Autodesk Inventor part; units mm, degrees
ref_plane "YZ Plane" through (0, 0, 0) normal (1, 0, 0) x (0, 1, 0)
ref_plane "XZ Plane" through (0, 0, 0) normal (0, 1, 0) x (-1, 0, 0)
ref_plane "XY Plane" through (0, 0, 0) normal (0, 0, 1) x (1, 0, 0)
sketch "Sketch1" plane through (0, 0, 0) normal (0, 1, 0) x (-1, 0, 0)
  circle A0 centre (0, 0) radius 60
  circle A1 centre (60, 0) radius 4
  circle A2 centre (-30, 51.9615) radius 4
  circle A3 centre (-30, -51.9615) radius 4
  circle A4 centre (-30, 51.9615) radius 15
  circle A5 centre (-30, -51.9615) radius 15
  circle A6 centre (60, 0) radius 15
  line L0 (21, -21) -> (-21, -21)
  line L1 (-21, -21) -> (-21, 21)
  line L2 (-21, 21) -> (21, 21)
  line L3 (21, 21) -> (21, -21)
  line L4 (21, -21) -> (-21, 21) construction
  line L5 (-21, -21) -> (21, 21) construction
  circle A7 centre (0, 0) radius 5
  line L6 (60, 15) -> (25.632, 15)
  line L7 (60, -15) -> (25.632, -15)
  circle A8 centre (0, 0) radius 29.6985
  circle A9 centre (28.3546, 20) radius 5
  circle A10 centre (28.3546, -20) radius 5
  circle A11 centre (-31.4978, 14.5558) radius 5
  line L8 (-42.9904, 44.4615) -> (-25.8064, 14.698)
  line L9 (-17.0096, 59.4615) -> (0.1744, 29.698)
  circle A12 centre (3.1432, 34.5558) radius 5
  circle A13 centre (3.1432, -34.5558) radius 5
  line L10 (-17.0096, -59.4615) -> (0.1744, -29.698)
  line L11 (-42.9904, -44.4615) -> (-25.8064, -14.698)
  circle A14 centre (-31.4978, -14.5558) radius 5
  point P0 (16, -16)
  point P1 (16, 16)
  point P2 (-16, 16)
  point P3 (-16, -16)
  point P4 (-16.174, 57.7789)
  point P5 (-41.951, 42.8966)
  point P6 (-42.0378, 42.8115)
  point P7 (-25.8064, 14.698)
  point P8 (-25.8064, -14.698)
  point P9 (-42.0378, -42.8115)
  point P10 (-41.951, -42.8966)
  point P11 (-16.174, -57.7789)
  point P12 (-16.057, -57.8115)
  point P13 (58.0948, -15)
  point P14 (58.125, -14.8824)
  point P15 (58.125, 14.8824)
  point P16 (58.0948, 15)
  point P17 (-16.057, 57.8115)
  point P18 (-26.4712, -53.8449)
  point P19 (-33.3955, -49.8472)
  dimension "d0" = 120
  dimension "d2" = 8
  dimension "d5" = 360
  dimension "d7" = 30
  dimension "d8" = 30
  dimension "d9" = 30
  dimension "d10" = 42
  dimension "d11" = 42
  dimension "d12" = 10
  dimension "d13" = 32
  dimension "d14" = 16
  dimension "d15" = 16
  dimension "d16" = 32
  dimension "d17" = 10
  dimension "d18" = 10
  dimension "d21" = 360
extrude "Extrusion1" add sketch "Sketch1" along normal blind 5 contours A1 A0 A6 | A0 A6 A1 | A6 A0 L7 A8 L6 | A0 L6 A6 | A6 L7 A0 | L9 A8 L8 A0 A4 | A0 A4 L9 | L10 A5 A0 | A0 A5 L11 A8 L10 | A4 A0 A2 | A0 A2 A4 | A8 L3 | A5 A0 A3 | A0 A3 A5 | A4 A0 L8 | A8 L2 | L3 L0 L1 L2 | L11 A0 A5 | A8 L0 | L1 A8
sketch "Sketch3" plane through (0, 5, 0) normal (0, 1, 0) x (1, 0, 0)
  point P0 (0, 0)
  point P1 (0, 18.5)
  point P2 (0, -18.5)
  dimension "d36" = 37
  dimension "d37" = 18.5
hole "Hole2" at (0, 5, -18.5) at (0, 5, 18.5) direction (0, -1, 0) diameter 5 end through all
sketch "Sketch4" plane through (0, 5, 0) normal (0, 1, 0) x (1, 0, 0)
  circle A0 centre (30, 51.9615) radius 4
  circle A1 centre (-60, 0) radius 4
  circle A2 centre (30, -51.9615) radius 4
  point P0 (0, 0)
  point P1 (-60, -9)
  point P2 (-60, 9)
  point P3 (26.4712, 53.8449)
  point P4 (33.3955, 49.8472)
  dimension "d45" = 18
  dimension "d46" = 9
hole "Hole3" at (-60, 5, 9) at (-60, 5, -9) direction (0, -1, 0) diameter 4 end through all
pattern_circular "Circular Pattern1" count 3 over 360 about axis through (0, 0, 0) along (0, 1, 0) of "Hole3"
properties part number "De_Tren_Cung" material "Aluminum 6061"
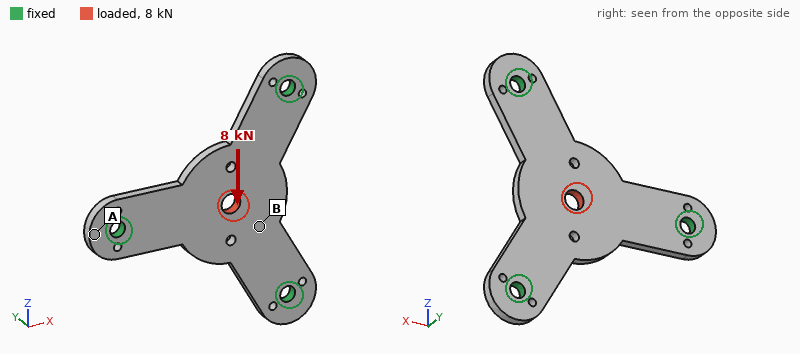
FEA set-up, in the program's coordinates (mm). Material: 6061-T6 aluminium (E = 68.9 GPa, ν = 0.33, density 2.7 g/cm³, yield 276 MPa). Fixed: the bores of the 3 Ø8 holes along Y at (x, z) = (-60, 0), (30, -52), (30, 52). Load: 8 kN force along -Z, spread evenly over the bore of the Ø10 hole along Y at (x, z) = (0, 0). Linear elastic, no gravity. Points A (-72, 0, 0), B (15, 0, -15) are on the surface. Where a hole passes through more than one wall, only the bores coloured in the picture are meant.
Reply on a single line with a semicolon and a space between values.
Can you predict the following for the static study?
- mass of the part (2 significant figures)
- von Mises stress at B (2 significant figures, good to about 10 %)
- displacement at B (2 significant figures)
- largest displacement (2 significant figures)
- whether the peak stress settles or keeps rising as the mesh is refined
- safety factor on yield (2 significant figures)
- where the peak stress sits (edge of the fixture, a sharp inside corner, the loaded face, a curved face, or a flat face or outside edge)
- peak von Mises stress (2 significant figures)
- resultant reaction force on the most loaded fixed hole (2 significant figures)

85 g; 30 MPa; 20 µm; 40 µm; settles; 2.8; the loaded face; 98 MPa; 4.1 kN
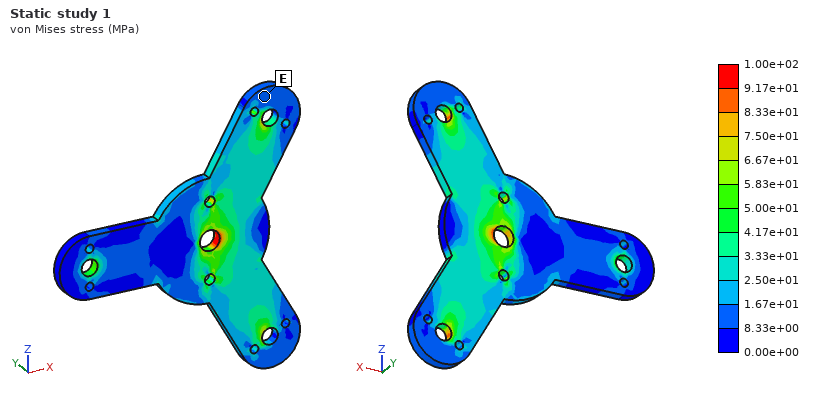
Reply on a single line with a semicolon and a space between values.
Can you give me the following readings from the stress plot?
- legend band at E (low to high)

8.33e+00 to 1.67e+01 MPa
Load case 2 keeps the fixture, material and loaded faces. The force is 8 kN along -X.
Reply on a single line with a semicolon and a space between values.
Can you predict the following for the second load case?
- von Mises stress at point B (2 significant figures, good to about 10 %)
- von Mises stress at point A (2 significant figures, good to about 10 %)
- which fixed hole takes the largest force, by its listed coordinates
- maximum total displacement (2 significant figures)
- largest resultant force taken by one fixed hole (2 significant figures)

21 MPa; 11 MPa; (-60, 0); 39 µm; 4.7 kN
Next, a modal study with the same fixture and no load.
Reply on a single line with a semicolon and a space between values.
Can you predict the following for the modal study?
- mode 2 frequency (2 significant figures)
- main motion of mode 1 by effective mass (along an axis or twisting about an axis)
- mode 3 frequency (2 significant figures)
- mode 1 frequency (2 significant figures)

4300 Hz; along Y; 4300 Hz; 2200 Hz
